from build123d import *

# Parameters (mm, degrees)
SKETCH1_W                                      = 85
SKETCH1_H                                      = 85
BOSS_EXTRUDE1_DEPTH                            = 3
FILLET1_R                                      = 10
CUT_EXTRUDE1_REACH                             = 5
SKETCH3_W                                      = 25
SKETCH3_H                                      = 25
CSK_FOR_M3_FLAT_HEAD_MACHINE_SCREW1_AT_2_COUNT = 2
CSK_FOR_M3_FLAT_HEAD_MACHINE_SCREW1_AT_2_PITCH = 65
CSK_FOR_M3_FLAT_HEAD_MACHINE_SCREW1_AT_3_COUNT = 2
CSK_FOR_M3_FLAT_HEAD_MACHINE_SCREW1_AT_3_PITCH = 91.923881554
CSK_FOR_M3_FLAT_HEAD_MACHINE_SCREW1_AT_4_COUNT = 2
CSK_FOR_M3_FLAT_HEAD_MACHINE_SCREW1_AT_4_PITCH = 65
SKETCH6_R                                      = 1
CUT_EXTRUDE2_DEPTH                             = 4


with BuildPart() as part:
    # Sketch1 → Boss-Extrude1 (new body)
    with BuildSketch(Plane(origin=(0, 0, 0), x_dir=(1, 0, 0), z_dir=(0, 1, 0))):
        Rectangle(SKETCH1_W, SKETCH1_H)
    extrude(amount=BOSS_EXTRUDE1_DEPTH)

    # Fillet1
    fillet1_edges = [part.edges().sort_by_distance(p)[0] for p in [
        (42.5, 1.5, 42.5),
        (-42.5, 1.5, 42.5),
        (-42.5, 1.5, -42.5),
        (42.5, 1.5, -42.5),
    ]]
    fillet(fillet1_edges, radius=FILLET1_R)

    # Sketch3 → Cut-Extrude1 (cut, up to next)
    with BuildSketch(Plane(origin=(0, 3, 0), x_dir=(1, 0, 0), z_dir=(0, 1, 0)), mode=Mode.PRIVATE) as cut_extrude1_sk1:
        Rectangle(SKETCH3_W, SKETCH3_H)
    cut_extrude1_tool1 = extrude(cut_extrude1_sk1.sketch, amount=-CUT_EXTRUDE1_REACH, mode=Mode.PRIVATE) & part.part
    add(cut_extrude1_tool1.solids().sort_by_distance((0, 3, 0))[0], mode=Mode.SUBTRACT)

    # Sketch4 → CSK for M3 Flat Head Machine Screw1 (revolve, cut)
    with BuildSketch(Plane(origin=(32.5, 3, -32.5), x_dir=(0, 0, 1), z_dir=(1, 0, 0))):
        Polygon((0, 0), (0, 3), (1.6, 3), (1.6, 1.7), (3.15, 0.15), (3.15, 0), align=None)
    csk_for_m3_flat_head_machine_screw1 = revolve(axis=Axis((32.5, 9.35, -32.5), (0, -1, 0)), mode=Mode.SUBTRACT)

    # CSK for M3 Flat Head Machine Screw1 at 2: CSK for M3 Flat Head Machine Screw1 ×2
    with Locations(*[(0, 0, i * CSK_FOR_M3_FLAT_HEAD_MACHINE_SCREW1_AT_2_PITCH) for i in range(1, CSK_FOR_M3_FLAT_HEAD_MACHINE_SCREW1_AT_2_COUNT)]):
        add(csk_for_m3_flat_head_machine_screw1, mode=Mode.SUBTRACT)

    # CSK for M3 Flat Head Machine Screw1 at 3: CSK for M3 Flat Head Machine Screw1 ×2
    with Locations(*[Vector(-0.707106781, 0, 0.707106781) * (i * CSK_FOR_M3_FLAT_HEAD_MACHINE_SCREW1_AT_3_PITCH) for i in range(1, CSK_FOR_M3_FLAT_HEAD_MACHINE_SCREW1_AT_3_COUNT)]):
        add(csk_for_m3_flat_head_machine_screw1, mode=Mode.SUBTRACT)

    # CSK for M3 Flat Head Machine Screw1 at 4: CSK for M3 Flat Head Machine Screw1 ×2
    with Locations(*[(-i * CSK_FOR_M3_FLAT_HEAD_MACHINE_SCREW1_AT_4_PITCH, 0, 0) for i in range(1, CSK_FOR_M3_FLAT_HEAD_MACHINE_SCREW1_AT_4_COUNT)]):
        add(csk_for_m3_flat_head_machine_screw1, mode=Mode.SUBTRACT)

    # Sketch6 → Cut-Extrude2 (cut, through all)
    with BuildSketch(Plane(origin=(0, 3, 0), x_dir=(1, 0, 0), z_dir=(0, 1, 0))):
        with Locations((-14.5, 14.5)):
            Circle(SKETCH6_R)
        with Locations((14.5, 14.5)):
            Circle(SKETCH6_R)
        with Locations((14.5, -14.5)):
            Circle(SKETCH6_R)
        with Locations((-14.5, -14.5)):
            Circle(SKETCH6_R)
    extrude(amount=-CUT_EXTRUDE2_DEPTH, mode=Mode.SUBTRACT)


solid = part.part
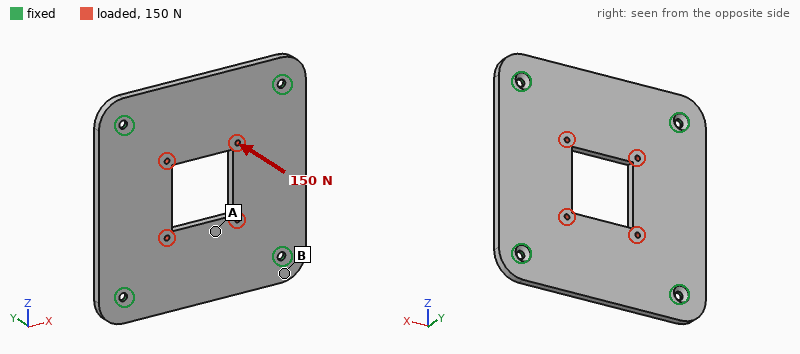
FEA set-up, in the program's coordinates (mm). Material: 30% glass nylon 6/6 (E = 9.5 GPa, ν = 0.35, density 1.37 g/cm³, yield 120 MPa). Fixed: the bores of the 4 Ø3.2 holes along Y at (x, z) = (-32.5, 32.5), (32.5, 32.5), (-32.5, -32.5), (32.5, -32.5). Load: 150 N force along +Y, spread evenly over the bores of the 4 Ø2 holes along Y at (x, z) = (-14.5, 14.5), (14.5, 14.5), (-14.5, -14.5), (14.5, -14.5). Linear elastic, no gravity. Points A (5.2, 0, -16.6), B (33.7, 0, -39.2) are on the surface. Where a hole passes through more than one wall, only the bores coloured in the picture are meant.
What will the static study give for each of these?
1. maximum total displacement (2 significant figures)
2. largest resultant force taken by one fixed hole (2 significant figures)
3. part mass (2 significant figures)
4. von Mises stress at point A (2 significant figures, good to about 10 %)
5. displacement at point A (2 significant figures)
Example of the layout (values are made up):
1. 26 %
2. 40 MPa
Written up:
1. 0.41 mm
2. 100 N
3. 26 g
4. 7.7 MPa
5. 0.35 mm
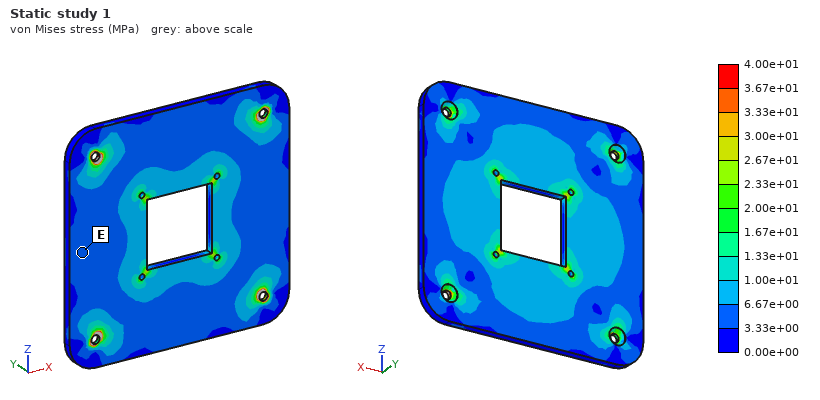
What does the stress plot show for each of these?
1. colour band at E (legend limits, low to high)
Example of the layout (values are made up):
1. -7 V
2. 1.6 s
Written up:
1. 3.33e+00 to 6.67e+00 MPa
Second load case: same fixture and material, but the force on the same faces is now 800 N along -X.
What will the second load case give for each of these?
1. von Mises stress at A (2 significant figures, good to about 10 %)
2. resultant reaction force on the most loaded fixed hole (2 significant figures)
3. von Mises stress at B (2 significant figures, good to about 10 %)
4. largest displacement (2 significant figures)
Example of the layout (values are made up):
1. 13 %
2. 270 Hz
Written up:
1. 2.8 MPa
2. 210 N
3. 2.4 MPa
4. 22 µm
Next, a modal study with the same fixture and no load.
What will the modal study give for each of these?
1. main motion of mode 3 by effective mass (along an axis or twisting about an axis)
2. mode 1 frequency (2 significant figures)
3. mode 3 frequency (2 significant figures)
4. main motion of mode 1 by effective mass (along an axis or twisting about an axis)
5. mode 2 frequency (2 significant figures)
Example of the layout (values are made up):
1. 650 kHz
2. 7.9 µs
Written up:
1. twisting about Z
2. 1100 Hz
3. 1700 Hz
4. along Y
5. 1600 Hz
